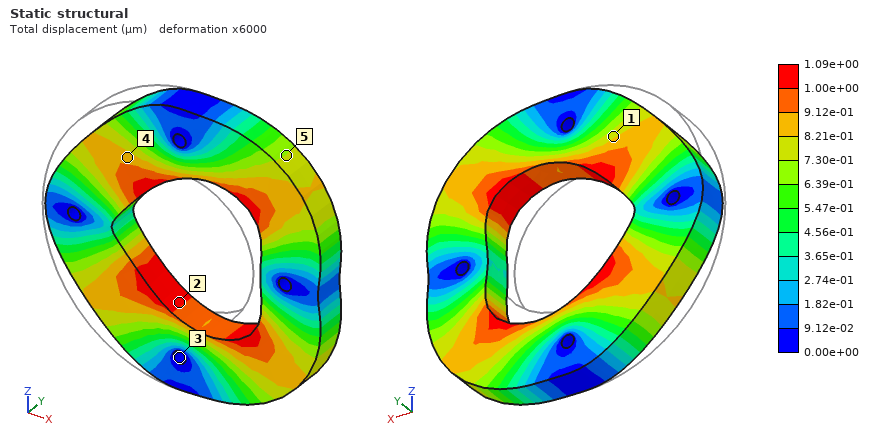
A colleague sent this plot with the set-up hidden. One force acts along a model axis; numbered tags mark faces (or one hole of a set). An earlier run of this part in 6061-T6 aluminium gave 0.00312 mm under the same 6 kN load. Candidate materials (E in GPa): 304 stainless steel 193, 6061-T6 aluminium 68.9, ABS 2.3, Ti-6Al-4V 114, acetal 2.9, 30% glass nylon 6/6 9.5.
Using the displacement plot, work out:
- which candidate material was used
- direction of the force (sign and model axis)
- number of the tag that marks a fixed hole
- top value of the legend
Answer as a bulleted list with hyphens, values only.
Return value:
- 304 stainless steel
- +X
- 3
- 1.09e+00 µm
